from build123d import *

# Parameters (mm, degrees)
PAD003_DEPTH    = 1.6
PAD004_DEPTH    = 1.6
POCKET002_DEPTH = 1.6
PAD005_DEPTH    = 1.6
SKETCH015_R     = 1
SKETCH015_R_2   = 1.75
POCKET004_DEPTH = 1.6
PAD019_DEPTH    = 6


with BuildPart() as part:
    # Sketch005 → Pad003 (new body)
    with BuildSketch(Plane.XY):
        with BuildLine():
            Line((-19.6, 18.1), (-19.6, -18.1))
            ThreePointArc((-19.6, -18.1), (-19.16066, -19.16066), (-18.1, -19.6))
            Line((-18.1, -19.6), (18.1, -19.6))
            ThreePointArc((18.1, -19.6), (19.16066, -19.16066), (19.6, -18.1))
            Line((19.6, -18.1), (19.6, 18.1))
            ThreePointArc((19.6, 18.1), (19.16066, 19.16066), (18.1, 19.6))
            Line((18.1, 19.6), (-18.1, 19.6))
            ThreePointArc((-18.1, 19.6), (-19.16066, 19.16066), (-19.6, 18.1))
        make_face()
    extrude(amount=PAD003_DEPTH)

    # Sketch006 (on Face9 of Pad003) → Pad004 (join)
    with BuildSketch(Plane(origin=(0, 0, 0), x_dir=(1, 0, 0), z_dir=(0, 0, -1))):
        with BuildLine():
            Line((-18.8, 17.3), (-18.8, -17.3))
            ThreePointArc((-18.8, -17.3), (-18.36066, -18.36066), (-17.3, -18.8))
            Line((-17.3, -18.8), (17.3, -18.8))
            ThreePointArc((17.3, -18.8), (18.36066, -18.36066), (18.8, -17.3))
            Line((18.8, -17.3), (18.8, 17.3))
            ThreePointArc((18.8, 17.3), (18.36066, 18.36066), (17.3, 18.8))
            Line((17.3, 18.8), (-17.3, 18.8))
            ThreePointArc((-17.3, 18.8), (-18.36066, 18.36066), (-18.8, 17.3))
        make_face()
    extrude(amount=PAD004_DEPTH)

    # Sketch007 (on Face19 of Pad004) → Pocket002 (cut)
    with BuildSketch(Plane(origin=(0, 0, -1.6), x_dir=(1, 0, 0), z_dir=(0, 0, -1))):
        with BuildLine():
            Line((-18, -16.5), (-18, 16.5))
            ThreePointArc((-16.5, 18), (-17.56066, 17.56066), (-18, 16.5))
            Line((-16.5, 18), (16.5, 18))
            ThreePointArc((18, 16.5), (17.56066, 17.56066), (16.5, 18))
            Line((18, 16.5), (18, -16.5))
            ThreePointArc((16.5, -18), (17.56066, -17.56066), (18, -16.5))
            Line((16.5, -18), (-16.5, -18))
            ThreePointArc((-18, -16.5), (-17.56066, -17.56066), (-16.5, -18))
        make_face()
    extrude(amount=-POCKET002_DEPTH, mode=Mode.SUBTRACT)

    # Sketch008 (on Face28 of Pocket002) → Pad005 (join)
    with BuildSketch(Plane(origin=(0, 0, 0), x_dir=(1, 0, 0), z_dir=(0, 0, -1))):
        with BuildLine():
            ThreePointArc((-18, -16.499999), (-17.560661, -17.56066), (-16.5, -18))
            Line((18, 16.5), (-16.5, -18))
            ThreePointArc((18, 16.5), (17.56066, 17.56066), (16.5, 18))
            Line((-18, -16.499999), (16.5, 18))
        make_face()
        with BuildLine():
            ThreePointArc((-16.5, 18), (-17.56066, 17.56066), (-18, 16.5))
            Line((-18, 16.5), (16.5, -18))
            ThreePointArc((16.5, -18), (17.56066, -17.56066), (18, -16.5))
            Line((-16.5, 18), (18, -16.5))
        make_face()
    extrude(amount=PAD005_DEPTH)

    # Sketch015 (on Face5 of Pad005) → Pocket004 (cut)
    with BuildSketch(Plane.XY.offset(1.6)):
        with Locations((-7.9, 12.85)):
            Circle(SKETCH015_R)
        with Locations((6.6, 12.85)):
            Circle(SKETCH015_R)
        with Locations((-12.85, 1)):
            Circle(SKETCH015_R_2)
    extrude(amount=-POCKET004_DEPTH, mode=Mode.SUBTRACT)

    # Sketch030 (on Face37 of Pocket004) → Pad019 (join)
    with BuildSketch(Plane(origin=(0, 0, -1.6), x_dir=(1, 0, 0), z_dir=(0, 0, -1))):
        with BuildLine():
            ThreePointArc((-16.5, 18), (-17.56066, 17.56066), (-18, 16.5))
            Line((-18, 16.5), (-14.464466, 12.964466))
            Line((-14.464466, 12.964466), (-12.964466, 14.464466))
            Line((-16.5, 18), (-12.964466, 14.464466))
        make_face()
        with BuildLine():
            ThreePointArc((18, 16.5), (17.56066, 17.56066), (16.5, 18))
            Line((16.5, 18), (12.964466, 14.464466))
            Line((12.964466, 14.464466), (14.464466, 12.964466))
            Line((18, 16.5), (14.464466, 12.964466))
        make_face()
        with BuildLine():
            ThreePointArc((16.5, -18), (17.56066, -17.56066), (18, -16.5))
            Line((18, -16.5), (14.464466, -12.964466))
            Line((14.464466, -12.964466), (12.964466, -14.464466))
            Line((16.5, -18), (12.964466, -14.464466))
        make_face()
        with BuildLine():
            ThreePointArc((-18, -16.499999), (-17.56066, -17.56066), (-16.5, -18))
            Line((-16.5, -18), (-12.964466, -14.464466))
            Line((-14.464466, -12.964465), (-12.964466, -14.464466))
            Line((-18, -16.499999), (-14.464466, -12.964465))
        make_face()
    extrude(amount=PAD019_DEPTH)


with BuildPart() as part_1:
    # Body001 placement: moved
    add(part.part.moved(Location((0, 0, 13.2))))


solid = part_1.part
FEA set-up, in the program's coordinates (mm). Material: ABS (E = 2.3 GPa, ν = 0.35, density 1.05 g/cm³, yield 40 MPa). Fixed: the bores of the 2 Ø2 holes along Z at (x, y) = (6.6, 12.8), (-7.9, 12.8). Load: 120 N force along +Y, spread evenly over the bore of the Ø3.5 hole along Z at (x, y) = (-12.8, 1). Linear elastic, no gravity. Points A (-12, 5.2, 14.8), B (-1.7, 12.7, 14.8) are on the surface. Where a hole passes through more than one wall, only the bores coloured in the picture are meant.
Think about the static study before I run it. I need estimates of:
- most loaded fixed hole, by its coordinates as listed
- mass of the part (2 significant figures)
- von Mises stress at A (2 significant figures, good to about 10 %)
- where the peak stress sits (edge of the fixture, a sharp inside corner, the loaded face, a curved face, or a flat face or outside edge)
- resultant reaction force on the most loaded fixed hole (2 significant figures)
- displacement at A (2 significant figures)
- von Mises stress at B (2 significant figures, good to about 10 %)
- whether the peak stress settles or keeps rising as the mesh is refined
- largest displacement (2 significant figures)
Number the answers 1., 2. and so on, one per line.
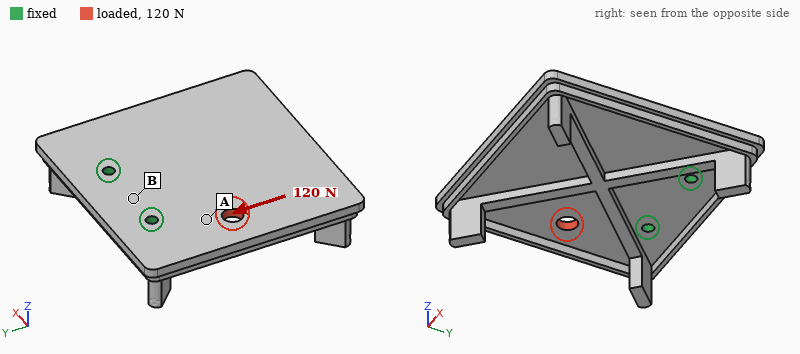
1. (-7.9, 12.8)
2. 3.4 g
3. 7.7 MPa
4. edge of the fixture
5. 150 N
6. 0.057 mm
7. 2.1 MPa
8. keeps rising
9. 0.14 mm
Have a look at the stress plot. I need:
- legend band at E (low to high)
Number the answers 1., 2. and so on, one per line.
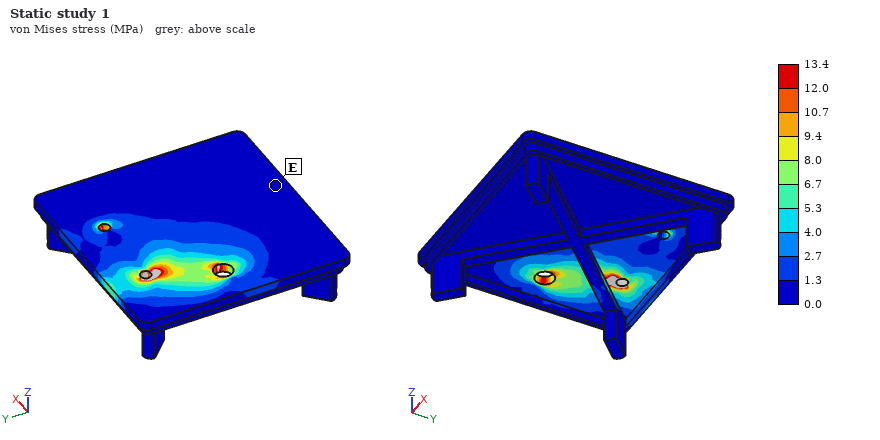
1. 0.0 to 1.3 MPa
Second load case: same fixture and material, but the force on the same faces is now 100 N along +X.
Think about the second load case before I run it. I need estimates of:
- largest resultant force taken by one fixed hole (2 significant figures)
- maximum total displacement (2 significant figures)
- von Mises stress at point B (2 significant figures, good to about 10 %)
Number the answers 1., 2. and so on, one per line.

1. 94 N
2. 0.14 mm
3. 3.5 MPa
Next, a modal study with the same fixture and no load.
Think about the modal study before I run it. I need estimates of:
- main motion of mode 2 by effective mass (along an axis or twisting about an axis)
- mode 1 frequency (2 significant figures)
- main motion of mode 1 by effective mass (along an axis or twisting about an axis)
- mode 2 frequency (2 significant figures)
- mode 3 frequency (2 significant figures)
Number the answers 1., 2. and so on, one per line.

1. twisting about Y
2. 360 Hz
3. along Z
4. 710 Hz
5. 1800 Hz
